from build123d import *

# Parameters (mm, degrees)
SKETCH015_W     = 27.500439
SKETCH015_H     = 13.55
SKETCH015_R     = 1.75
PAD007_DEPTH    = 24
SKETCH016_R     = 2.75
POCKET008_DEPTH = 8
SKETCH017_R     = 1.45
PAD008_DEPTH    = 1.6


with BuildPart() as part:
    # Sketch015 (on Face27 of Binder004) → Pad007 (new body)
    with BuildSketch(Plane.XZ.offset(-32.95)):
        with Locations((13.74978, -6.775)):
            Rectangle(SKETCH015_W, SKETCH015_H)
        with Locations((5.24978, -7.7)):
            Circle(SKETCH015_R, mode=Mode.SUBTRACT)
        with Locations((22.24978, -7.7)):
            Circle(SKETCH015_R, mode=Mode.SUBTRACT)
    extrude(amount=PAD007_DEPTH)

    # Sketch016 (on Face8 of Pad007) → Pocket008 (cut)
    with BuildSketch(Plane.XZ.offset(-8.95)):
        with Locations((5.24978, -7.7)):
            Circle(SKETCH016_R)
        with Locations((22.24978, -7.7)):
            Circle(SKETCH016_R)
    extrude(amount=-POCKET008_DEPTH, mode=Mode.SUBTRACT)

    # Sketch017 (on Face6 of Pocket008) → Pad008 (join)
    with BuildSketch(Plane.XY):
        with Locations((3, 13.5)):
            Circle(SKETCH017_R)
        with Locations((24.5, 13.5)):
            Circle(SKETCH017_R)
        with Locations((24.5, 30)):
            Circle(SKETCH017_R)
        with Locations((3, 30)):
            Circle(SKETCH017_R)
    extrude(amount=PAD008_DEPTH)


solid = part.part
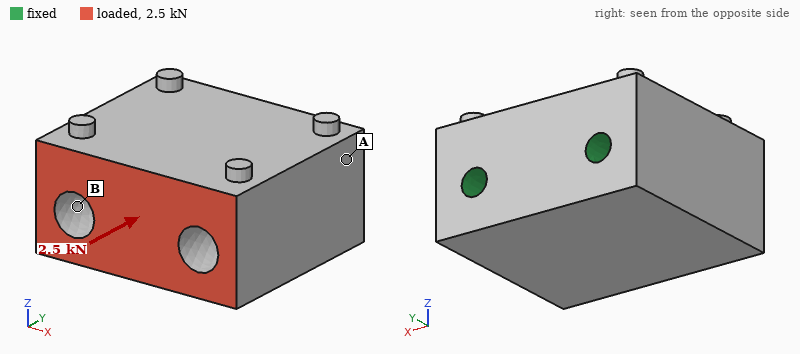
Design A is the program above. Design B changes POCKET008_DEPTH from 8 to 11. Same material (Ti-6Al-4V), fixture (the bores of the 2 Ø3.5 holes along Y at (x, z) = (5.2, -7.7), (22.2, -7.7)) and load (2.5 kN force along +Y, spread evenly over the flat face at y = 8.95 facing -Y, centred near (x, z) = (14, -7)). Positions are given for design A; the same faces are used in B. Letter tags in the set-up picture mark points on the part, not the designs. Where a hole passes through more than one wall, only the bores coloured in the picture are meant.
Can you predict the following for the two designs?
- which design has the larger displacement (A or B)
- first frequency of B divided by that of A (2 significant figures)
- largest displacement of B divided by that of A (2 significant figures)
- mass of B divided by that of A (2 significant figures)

B
0.72
1.2
0.99
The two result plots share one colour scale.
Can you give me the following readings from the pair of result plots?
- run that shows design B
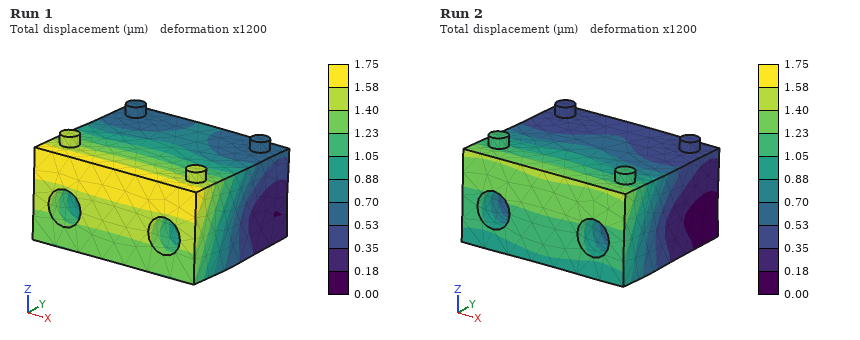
Run 1
